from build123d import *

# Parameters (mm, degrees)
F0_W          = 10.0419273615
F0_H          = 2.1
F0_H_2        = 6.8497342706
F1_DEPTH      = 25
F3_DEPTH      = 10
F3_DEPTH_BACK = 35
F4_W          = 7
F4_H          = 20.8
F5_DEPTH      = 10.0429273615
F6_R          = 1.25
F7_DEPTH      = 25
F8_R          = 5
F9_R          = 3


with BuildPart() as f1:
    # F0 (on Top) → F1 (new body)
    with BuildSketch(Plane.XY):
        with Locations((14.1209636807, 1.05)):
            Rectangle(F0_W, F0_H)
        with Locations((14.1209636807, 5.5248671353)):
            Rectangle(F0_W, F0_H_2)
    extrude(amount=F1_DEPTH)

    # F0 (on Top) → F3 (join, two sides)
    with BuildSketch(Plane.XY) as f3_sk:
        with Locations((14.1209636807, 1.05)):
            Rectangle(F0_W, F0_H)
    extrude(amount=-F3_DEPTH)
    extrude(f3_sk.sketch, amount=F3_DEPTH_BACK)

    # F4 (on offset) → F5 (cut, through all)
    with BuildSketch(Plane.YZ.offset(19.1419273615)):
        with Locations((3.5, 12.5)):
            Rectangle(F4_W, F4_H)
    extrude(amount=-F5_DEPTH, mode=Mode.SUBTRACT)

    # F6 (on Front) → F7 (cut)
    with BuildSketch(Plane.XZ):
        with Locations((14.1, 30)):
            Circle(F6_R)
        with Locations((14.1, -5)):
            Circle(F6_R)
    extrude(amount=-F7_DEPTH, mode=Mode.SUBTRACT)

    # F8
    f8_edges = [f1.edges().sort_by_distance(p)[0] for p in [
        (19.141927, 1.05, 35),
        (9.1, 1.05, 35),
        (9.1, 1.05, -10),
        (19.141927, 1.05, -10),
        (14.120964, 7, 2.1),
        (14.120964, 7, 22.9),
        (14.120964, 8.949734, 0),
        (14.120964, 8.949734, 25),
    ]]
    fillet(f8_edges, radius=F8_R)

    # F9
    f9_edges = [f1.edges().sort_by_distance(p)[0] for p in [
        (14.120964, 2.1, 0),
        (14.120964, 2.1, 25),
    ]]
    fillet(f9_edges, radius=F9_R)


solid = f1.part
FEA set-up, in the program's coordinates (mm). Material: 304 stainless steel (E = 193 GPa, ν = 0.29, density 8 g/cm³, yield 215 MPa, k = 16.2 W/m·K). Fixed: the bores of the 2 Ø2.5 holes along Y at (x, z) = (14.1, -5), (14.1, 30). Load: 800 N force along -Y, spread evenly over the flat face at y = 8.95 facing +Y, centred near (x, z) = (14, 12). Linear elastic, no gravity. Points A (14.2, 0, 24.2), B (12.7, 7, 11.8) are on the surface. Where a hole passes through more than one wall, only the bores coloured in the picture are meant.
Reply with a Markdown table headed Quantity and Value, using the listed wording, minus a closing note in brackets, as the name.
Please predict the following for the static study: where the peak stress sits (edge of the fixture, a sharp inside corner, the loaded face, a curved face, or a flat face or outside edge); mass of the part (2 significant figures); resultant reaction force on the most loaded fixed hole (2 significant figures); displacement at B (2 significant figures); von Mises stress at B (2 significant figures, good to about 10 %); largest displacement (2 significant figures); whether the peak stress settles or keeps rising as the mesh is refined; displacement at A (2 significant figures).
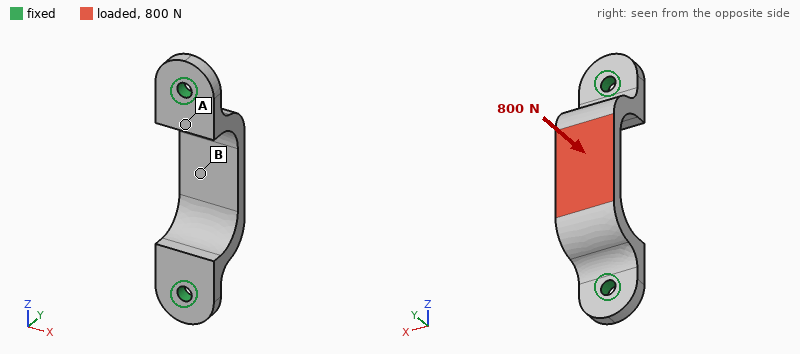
| Quantity | Value |
|---|---|
| where the peak stress sits | edge of the fixture |
| mass of the part | 9.4 g |
| resultant reaction force on the most loaded fixed hole | 690 N |
| displacement at B | 17 µm |
| von Mises stress at B | 68 MPa |
| largest displacement | 19 µm |
| whether the peak stress settles or keeps rising as the mesh is refined | keeps rising |
| displacement at A | 3.6 µm |
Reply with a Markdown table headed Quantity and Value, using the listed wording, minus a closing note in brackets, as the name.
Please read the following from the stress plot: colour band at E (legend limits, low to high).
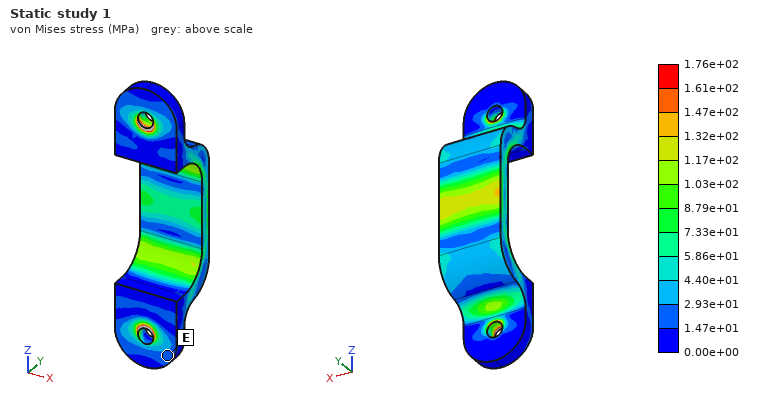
| Quantity | Value |
|---|---|
| colour band at E | 1.47e+01 to 2.93e+01 MPa |
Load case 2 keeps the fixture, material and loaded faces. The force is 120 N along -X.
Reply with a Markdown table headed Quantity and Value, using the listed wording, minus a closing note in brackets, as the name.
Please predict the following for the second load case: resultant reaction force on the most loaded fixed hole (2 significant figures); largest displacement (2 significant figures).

| Quantity | Value |
|---|---|
| resultant reaction force on the most loaded fixed hole | 60 N |
| largest displacement | 8.8 µm |
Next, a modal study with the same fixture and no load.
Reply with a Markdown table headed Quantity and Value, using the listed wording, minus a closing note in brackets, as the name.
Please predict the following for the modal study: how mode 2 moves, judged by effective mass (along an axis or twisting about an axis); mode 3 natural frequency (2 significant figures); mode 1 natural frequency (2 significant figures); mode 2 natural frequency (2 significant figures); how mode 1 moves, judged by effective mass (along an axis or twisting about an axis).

| Quantity | Value |
|---|---|
| how mode 2 moves, judged by effective mass | along Z |
| mode 3 natural frequency | 20 kHz |
| mode 1 natural frequency | 10 kHz |
| mode 2 natural frequency | 15 kHz |
| how mode 1 moves, judged by effective mass | along X |
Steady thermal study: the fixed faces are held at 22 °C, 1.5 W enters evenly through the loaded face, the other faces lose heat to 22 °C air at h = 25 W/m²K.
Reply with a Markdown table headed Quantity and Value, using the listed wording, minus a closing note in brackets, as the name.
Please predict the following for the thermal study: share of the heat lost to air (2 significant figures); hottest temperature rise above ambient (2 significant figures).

| Quantity | Value |
|---|---|
| share of the heat lost to air | 22 % |
| hottest temperature rise above ambient | 28 K |
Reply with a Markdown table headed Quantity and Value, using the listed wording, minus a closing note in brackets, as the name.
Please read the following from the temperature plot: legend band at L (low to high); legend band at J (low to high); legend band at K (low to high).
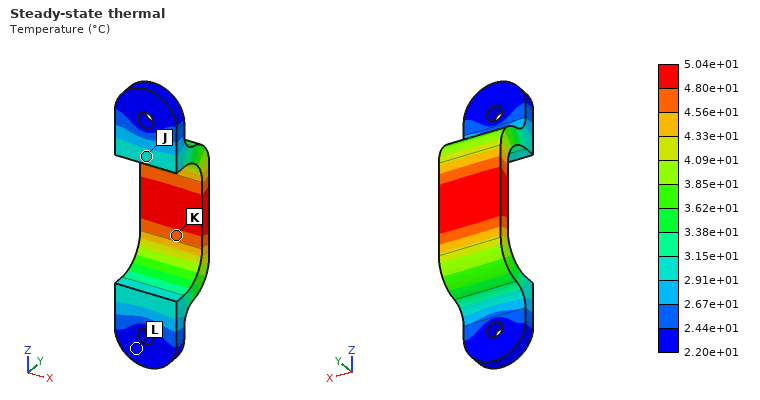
| Quantity | Value |
|---|---|
| legend band at L | 2.20e+01 to 2.44e+01 °C |
| legend band at J | 2.91e+01 to 3.15e+01 °C |
| legend band at K | 4.56e+01 to 4.80e+01 °C |
